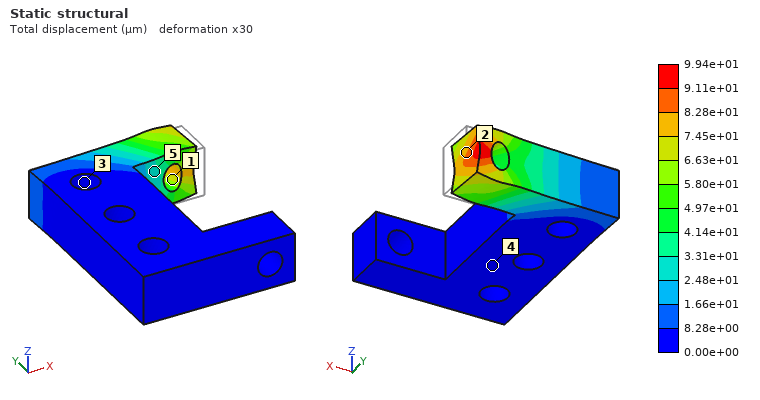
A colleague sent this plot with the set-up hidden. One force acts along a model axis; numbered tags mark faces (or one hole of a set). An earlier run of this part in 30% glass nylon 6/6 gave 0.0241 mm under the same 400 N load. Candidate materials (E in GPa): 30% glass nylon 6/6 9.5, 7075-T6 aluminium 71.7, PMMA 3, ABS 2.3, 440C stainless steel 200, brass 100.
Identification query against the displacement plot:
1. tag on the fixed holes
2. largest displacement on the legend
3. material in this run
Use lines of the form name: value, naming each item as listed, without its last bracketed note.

tag on the fixed holes: 3
largest displacement on the legend: 9.94e+01 µm
material in this run: ABS
